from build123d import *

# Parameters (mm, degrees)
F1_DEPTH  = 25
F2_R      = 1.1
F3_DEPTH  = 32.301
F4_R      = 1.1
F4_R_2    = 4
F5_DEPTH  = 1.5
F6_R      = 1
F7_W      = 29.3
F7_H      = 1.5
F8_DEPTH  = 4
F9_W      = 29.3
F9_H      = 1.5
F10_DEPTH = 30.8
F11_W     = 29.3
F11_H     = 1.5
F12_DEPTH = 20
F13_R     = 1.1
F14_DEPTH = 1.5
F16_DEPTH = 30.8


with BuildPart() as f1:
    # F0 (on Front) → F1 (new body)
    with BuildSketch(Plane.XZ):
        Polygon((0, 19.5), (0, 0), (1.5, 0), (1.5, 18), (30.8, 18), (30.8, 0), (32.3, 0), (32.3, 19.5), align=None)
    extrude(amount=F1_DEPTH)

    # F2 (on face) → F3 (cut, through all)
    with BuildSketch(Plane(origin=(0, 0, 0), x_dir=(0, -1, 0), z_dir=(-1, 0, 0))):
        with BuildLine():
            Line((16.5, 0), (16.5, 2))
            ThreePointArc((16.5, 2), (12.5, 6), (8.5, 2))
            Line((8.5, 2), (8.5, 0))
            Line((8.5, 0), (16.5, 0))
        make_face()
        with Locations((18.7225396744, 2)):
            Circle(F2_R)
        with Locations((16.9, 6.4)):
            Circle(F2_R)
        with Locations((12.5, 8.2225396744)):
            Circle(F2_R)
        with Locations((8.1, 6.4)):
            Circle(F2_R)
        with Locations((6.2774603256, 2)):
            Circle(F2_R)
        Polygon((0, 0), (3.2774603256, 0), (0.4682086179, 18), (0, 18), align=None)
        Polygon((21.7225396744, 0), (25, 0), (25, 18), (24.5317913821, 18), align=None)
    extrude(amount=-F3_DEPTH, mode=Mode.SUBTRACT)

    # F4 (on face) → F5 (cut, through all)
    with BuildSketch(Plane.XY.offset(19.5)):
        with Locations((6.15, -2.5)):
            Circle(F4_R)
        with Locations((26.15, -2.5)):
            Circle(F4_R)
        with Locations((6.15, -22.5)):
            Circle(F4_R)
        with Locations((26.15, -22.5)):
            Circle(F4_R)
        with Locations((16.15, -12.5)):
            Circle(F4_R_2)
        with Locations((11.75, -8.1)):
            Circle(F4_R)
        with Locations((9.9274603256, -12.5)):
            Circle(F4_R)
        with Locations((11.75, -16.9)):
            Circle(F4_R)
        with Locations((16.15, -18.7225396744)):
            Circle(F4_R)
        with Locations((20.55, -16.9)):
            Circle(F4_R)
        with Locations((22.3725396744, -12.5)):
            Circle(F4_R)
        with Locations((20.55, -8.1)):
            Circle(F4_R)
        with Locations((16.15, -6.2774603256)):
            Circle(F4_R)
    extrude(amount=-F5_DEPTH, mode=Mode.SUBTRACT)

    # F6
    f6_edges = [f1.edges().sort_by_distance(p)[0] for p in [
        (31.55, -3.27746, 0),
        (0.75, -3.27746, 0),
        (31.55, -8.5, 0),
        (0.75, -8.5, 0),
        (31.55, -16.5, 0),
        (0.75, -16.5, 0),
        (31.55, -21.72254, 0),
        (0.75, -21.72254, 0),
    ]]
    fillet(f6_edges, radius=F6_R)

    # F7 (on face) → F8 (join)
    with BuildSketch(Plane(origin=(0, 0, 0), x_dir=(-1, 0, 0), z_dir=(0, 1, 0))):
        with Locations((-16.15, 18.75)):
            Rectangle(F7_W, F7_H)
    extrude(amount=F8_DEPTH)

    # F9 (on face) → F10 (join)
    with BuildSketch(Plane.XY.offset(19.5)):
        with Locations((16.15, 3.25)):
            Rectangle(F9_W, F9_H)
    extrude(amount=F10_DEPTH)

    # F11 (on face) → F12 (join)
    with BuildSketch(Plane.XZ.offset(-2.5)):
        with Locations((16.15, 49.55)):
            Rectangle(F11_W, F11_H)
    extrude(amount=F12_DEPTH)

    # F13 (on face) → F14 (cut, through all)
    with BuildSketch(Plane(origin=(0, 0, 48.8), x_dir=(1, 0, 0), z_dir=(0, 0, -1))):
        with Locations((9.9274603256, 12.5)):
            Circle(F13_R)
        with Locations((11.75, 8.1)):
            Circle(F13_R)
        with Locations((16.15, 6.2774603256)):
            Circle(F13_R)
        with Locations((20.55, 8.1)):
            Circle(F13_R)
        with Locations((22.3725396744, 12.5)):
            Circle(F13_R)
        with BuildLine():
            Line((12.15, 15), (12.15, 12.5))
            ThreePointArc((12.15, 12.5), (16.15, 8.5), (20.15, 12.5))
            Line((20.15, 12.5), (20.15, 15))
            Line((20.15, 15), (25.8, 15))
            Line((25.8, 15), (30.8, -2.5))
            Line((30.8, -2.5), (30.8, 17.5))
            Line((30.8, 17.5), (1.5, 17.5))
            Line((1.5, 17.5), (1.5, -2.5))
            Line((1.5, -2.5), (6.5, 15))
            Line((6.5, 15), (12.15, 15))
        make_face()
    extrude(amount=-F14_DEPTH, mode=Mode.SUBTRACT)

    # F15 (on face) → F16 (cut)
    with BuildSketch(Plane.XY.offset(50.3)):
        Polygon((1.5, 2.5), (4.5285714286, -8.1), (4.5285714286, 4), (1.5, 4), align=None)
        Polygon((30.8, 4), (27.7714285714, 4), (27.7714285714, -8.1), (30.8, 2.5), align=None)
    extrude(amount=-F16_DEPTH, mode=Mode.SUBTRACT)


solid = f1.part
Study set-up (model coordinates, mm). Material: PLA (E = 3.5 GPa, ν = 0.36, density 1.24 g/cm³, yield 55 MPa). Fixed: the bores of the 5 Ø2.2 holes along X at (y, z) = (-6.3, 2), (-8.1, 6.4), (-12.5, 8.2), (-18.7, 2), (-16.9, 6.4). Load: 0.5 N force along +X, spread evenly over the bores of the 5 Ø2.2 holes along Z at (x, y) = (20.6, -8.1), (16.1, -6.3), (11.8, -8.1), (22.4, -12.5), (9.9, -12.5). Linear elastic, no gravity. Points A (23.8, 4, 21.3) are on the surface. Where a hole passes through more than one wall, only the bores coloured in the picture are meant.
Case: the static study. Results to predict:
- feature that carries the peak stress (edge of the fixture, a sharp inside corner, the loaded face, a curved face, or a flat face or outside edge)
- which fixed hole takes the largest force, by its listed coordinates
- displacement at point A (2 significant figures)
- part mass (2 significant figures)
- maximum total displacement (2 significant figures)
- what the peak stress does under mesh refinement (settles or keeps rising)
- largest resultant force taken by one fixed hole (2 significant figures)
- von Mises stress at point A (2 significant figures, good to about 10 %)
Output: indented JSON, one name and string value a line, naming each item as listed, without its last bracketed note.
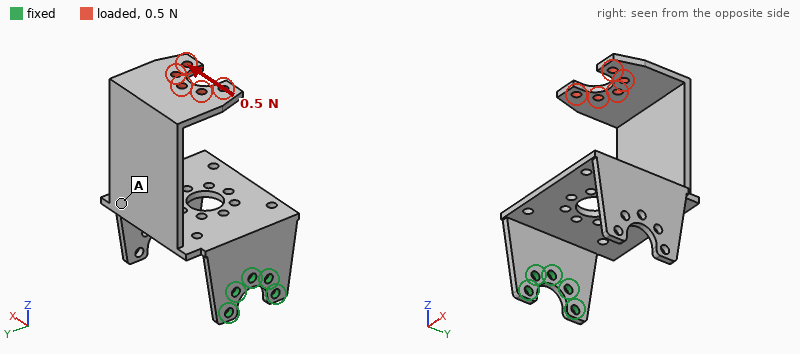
{
  "feature that carries the peak stress": "edge of the fixture",
  "which fixed hole takes the largest force, by its listed coordinates": "(-12.5, 8.2)",
  "displacement at point A": "0.38 mm",
  "part mass": "4.7 g",
  "maximum total displacement": "0.76 mm",
  "what the peak stress does under mesh refinement": "keeps rising",
  "largest resultant force taken by one fixed hole": "1.9 N",
  "von Mises stress at point A": "0.61 MPa"
}
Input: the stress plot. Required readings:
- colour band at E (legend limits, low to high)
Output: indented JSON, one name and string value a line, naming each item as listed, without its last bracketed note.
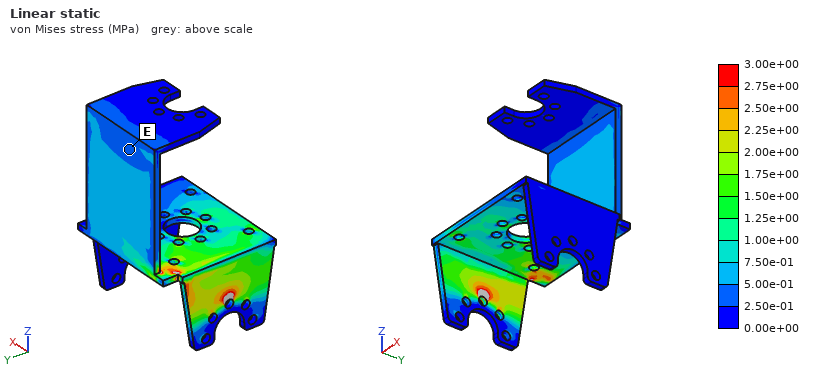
{
  "colour band at E": "2.50e-01 to 5.00e-01 MPa"
}
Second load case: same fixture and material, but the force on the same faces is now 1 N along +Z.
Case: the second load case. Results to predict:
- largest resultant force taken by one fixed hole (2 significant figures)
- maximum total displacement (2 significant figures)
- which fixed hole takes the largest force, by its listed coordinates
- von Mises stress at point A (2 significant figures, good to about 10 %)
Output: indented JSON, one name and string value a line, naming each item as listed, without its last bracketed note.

{
  "largest resultant force taken by one fixed hole": "1.4 N",
  "maximum total displacement": "0.78 mm",
  "which fixed hole takes the largest force, by its listed coordinates": "(-12.5, 8.2)",
  "von Mises stress at point A": "1.2 MPa"
}
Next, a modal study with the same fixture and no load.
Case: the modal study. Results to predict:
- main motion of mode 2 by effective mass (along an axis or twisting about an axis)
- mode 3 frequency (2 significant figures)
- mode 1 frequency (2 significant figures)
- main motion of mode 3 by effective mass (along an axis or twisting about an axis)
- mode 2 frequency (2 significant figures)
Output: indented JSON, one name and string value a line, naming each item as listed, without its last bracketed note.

{
  "main motion of mode 2 by effective mass": "along Y",
  "mode 3 frequency": "270 Hz",
  "mode 1 frequency": "100 Hz",
  "main motion of mode 3 by effective mass": "along Y",
  "mode 2 frequency": "170 Hz"
}
